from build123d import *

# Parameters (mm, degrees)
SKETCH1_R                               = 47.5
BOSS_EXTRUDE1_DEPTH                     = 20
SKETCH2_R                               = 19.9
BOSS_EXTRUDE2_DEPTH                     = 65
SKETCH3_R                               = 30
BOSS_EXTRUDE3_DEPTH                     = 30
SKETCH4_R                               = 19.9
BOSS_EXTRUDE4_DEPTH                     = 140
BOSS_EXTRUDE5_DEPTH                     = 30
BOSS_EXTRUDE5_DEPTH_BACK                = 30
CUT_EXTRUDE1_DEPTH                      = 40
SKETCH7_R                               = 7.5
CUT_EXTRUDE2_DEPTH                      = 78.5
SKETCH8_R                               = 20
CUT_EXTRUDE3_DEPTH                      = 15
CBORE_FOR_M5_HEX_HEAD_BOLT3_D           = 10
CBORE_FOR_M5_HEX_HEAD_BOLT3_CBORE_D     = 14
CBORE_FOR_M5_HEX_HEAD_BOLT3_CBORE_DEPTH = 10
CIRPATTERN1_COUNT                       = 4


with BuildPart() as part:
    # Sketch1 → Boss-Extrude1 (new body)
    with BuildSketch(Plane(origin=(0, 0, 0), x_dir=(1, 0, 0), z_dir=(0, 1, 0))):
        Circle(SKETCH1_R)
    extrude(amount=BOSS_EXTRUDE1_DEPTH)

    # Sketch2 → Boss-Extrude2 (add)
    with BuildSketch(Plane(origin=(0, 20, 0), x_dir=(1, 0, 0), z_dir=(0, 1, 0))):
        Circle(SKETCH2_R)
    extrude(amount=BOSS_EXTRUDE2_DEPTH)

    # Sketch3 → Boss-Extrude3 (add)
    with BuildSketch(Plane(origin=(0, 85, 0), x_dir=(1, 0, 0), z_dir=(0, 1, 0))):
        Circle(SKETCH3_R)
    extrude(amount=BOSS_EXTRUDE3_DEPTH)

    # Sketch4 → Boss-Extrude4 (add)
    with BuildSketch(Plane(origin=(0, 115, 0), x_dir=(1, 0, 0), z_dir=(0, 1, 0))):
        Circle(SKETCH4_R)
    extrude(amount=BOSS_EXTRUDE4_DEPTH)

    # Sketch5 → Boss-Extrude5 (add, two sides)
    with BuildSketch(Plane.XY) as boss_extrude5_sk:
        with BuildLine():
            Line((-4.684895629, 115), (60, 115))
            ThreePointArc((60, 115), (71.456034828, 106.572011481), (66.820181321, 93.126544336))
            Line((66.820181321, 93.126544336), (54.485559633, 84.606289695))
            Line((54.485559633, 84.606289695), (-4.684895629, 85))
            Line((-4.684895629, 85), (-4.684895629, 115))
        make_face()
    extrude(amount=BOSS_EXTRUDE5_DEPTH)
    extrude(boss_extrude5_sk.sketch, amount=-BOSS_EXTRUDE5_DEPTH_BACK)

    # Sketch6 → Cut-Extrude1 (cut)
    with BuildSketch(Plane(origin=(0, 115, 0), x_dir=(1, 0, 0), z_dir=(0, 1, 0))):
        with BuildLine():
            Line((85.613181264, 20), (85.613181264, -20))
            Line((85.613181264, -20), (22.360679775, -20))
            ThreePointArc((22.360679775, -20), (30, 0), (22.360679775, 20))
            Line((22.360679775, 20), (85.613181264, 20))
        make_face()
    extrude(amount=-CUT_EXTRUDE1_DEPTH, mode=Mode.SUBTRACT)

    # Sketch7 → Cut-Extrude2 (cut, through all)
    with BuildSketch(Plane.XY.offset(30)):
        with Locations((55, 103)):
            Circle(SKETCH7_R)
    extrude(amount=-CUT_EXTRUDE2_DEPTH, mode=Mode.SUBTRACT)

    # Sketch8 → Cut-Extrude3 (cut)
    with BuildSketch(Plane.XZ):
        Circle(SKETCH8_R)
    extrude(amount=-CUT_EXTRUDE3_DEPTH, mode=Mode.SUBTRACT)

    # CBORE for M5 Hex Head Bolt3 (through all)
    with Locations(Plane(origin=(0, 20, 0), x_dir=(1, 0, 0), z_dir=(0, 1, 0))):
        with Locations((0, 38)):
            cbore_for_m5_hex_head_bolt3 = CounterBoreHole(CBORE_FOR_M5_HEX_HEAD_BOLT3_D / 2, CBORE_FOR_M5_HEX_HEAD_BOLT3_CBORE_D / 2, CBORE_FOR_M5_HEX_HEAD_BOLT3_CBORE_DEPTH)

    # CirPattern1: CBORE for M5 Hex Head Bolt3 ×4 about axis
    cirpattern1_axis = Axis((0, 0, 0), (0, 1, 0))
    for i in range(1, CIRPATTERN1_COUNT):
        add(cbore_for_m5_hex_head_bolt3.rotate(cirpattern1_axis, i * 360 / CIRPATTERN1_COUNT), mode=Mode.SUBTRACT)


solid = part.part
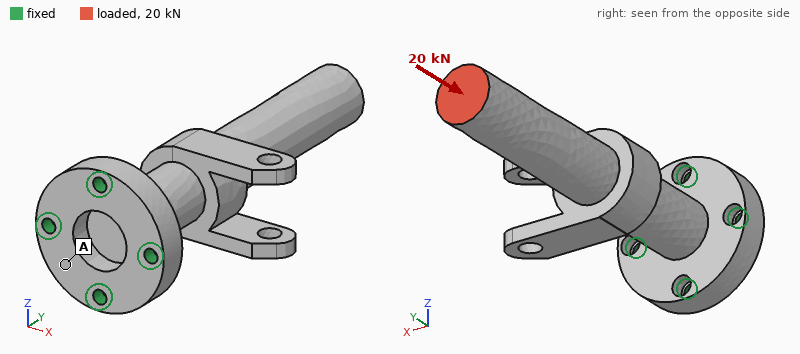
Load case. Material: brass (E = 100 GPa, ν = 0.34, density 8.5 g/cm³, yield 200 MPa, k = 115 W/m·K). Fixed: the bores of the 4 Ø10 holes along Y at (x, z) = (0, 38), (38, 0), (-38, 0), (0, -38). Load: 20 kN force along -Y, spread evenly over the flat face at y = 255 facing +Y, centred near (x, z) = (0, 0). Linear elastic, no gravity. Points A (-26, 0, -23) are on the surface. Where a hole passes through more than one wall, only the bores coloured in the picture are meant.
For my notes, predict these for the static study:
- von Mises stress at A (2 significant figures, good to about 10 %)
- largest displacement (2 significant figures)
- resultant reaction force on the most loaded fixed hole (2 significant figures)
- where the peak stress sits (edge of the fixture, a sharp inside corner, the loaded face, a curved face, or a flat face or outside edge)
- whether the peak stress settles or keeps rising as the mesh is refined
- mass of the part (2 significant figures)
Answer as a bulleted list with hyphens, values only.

- 11 MPa
- 48 µm
- 6.2 kN
- edge of the fixture
- keeps rising
- 4.1 kg
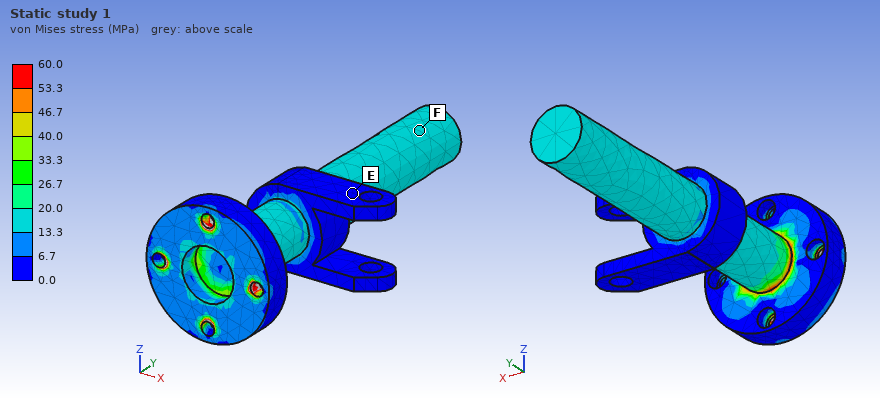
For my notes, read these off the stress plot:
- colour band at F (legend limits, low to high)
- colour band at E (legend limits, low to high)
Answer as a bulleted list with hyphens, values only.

- 13.3 to 20.0 MPa
- 0.0 to 6.7 MPa
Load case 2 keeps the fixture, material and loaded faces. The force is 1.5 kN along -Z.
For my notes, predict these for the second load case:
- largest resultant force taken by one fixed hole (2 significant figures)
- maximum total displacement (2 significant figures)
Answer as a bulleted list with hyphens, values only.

- 5.9 kN
- 0.68 mm
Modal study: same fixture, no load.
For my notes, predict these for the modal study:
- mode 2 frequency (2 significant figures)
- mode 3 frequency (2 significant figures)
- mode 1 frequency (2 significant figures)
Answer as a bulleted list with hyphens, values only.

- 280 Hz
- 1300 Hz
- 280 Hz
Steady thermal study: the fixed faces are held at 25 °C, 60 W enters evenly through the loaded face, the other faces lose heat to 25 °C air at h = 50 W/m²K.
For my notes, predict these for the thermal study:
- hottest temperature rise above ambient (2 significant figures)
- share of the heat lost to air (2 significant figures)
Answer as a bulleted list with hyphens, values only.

- 57 K
- 72 %
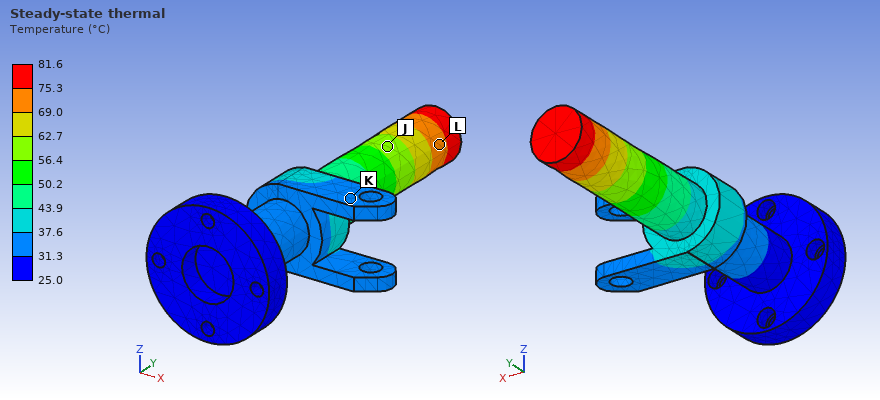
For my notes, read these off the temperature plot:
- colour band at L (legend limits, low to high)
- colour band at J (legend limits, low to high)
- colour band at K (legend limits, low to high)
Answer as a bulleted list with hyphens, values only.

- 69.0 to 75.3 °C
- 56.4 to 62.7 °C
- 31.3 to 37.6 °C
